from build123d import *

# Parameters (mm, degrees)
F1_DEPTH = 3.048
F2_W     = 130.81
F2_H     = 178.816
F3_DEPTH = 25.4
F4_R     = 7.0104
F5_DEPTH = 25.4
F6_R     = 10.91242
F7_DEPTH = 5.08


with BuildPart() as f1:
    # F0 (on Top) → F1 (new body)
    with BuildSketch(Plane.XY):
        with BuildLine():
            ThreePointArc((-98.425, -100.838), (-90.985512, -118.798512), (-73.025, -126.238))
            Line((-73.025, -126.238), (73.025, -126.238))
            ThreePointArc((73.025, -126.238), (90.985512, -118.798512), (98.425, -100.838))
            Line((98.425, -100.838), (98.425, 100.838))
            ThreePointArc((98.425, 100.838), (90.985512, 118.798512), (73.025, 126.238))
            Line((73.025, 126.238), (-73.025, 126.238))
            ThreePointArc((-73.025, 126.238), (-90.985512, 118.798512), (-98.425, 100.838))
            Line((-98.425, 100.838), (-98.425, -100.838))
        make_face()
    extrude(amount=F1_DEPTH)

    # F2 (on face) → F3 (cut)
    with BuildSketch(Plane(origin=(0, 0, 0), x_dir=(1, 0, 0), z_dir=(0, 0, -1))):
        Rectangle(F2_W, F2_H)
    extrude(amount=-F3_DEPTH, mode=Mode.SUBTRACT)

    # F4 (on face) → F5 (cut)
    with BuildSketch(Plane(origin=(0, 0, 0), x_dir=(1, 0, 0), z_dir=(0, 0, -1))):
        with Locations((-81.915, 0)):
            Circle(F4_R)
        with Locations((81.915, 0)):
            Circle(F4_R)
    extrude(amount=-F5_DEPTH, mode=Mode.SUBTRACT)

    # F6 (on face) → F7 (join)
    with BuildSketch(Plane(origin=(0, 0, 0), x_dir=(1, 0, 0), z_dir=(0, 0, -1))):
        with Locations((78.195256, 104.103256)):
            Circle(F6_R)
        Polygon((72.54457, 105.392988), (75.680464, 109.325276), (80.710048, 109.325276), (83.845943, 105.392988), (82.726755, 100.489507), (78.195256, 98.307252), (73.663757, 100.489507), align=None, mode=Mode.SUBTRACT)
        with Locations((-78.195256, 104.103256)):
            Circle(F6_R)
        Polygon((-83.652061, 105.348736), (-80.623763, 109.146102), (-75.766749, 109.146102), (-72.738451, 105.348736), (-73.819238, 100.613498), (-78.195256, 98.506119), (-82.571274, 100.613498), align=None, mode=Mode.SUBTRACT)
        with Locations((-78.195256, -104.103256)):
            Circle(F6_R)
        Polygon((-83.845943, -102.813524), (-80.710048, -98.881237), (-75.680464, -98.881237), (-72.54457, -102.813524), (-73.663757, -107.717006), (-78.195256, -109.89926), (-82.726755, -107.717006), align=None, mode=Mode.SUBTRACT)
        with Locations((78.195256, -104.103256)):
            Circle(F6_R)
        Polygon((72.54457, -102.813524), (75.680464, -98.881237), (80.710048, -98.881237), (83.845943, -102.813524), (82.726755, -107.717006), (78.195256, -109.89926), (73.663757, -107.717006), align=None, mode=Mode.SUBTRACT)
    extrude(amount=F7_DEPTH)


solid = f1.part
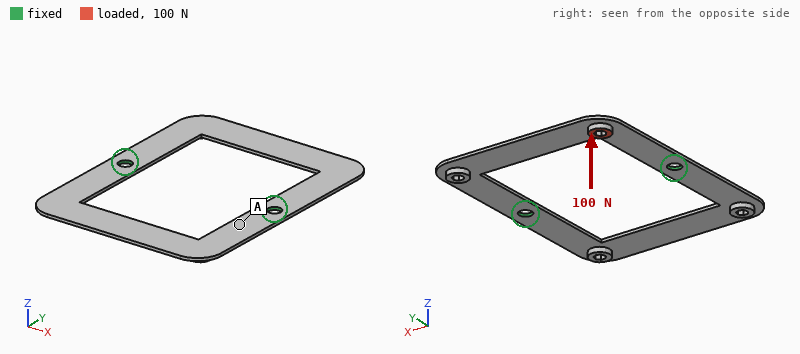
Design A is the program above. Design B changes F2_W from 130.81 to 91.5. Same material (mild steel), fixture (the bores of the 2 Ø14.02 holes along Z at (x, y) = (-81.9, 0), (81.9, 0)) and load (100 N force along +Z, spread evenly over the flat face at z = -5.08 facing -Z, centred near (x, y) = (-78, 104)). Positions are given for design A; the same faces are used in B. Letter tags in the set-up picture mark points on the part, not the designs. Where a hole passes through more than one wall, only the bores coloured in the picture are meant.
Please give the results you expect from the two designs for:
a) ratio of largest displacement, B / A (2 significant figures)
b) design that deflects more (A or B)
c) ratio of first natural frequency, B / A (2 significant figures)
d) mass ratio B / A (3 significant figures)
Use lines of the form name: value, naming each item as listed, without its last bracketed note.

ratio of largest displacement, B / A: 0.70
design that deflects more: A
ratio of first natural frequency, B / A: 1.2
mass ratio B / A: 1.26
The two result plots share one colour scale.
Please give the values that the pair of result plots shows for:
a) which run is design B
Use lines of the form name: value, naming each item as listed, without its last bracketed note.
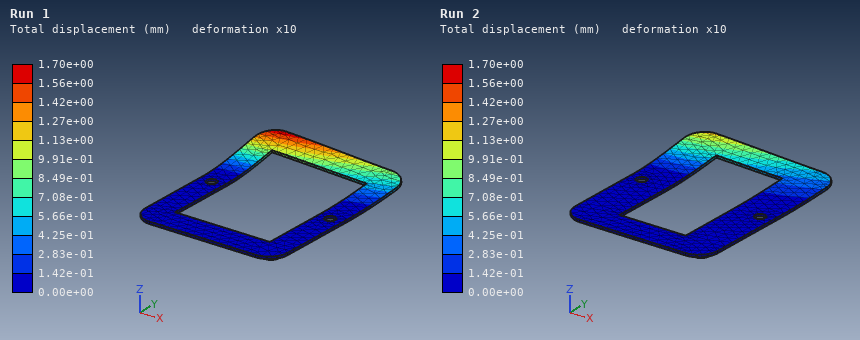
which run is design B: Run 2
